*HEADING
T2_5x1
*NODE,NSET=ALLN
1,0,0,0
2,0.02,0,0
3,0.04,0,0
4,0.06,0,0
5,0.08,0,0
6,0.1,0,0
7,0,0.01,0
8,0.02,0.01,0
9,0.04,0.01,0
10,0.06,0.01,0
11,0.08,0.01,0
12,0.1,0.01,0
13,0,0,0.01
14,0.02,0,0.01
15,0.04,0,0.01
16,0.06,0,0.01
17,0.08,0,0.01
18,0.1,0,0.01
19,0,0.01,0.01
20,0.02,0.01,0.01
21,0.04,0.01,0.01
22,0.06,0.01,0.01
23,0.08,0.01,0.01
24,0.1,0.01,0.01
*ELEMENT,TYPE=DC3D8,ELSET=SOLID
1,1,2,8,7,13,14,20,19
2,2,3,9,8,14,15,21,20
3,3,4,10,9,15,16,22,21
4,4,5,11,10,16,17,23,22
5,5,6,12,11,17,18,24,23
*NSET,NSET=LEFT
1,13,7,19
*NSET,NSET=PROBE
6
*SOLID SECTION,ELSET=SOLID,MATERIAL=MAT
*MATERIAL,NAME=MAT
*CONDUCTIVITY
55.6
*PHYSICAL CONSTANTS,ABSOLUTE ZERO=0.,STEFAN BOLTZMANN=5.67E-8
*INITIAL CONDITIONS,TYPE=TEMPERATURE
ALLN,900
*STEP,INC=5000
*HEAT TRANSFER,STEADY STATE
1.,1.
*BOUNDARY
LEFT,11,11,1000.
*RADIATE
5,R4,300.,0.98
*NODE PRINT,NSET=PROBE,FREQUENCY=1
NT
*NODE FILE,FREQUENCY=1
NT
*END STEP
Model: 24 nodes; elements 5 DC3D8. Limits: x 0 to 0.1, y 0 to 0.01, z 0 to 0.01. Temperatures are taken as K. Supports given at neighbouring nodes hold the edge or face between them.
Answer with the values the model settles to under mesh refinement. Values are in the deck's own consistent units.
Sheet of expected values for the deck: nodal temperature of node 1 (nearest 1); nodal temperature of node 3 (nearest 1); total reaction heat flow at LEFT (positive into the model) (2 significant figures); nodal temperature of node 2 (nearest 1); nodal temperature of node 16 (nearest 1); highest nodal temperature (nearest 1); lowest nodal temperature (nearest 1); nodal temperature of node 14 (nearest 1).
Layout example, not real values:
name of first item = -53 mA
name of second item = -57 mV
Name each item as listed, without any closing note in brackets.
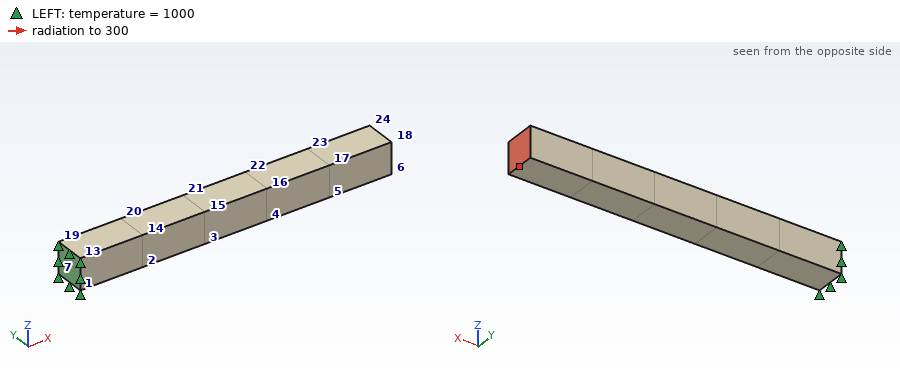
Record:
nodal temperature of node 1 = 1000 K
nodal temperature of node 3 = 971 K
total reaction heat flow at LEFT (positive into the model) = 4.1
nodal temperature of node 2 = 985 K
nodal temperature of node 16 = 956 K
highest nodal temperature = 1000 K
lowest nodal temperature = 927 K
nodal temperature of node 14 = 985 K
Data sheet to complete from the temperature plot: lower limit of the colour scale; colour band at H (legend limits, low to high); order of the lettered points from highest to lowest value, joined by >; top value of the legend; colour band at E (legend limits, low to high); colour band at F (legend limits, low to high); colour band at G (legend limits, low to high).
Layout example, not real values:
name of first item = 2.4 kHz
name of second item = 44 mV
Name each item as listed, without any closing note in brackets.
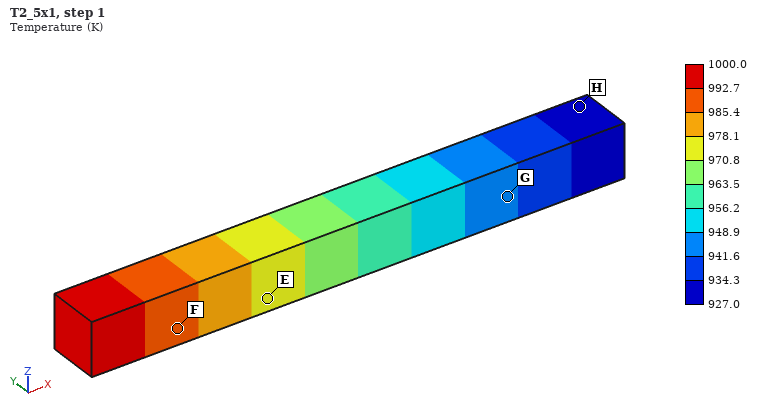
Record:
lower limit of the colour scale = 927.0 K
colour band at H = 927.0 to 934.3 K
order of the lettered points from highest to lowest value, joined by > = F > E > G > H
top value of the legend = 1000.0 K
colour band at E = 970.8 to 978.1 K
colour band at F = 985.4 to 992.7 K
colour band at G = 941.6 to 948.9 K
